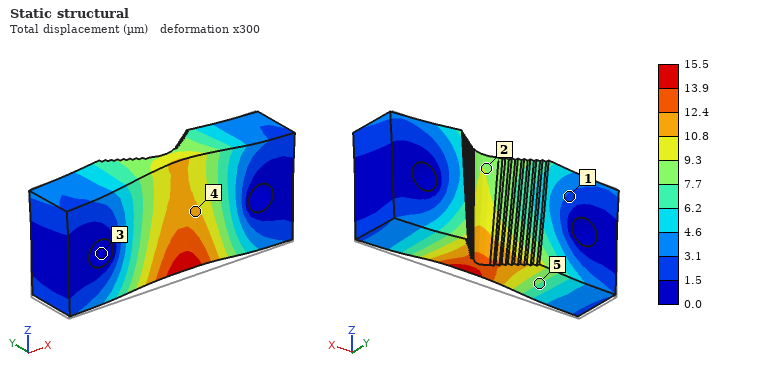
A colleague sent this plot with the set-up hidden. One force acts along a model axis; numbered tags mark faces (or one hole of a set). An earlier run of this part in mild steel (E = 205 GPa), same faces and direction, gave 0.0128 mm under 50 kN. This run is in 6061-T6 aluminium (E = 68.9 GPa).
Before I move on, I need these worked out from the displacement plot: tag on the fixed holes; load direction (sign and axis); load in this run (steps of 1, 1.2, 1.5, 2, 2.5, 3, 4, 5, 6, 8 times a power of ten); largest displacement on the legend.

3
+Z
20 kN
15.5 µm
